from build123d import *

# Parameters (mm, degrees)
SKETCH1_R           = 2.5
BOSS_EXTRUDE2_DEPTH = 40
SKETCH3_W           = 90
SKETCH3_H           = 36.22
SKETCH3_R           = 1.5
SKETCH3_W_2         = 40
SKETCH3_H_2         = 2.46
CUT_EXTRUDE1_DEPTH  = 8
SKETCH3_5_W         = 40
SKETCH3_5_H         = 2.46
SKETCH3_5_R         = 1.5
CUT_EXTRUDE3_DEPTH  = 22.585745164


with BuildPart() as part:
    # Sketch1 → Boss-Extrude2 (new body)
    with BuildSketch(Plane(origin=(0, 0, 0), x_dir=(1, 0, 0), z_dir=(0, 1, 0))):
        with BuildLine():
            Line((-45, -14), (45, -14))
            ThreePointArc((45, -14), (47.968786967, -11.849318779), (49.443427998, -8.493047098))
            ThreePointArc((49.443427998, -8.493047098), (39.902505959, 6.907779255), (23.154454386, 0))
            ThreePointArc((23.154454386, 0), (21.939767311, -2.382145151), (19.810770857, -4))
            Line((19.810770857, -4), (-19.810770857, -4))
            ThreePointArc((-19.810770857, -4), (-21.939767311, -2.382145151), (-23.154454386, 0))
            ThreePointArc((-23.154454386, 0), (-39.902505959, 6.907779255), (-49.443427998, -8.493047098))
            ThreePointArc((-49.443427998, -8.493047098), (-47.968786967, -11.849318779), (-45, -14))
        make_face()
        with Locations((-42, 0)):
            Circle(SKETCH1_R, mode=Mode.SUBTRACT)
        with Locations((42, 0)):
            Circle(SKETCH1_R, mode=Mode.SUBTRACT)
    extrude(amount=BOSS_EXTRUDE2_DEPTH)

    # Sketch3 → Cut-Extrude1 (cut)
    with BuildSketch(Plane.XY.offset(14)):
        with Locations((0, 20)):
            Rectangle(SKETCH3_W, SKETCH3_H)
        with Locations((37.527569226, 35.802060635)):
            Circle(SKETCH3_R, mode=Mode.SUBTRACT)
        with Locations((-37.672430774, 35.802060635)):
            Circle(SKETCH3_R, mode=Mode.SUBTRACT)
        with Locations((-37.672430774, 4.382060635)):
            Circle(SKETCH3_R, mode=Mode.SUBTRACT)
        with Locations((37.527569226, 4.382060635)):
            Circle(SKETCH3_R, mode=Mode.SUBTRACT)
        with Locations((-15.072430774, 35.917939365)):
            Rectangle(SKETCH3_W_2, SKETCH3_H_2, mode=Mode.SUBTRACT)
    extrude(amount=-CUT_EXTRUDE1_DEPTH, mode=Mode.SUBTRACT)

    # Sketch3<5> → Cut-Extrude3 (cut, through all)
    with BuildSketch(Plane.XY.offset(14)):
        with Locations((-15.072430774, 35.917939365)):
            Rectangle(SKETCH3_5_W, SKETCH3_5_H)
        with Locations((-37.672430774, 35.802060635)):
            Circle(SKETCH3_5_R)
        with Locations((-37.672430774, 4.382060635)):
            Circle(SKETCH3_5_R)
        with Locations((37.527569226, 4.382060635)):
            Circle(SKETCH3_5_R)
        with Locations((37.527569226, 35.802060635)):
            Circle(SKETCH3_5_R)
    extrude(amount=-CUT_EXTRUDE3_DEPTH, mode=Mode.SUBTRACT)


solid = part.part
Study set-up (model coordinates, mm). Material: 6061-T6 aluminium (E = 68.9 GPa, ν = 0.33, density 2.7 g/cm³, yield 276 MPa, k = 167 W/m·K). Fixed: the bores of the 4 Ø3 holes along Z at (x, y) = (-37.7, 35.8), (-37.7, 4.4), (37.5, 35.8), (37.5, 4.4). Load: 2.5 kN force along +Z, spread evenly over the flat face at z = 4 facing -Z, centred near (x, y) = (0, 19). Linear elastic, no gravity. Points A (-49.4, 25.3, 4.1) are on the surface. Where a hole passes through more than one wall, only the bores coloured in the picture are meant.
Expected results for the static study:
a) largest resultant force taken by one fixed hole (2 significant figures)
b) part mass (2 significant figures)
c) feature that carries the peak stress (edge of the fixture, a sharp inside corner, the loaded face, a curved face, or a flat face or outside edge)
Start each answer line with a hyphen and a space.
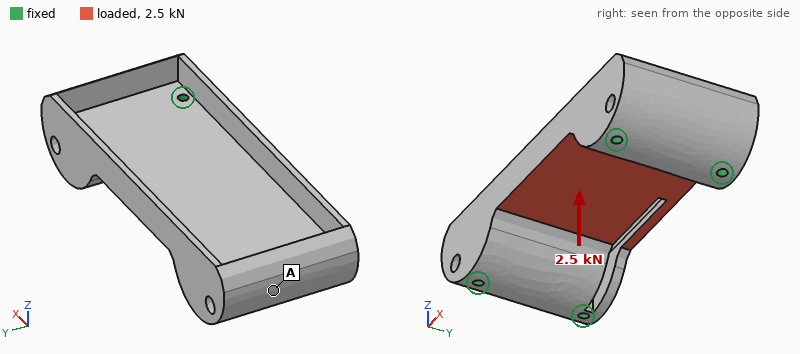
- 970 N
- 81 g
- a flat face or outside edge
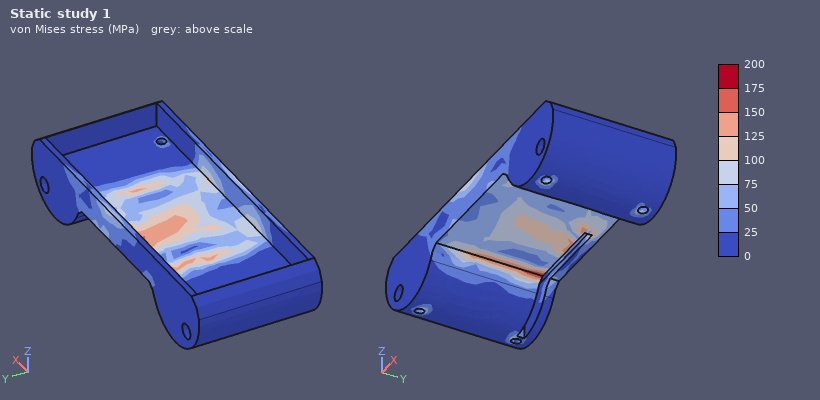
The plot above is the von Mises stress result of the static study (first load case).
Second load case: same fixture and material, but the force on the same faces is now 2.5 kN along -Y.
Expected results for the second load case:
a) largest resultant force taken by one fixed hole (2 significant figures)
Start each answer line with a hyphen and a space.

- 1.1 kN
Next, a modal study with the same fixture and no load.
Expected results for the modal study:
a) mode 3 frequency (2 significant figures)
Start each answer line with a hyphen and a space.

- 12 kHz
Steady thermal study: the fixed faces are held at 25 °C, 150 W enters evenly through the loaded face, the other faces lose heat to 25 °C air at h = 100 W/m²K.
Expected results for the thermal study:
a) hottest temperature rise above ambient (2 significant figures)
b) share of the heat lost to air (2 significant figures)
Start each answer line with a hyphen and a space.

- 76 K
- 15 %
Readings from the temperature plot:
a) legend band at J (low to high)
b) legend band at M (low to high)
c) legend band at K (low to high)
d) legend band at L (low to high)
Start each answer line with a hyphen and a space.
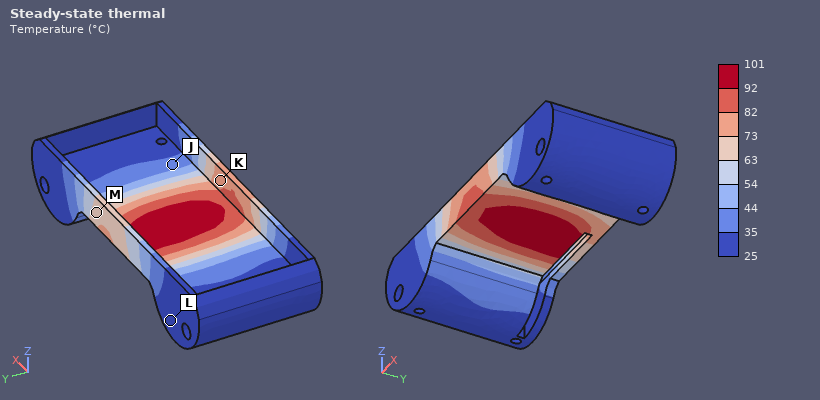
- 35 to 44 °C
- 63 to 73 °C
- 73 to 82 °C
- 25 to 35 °C
